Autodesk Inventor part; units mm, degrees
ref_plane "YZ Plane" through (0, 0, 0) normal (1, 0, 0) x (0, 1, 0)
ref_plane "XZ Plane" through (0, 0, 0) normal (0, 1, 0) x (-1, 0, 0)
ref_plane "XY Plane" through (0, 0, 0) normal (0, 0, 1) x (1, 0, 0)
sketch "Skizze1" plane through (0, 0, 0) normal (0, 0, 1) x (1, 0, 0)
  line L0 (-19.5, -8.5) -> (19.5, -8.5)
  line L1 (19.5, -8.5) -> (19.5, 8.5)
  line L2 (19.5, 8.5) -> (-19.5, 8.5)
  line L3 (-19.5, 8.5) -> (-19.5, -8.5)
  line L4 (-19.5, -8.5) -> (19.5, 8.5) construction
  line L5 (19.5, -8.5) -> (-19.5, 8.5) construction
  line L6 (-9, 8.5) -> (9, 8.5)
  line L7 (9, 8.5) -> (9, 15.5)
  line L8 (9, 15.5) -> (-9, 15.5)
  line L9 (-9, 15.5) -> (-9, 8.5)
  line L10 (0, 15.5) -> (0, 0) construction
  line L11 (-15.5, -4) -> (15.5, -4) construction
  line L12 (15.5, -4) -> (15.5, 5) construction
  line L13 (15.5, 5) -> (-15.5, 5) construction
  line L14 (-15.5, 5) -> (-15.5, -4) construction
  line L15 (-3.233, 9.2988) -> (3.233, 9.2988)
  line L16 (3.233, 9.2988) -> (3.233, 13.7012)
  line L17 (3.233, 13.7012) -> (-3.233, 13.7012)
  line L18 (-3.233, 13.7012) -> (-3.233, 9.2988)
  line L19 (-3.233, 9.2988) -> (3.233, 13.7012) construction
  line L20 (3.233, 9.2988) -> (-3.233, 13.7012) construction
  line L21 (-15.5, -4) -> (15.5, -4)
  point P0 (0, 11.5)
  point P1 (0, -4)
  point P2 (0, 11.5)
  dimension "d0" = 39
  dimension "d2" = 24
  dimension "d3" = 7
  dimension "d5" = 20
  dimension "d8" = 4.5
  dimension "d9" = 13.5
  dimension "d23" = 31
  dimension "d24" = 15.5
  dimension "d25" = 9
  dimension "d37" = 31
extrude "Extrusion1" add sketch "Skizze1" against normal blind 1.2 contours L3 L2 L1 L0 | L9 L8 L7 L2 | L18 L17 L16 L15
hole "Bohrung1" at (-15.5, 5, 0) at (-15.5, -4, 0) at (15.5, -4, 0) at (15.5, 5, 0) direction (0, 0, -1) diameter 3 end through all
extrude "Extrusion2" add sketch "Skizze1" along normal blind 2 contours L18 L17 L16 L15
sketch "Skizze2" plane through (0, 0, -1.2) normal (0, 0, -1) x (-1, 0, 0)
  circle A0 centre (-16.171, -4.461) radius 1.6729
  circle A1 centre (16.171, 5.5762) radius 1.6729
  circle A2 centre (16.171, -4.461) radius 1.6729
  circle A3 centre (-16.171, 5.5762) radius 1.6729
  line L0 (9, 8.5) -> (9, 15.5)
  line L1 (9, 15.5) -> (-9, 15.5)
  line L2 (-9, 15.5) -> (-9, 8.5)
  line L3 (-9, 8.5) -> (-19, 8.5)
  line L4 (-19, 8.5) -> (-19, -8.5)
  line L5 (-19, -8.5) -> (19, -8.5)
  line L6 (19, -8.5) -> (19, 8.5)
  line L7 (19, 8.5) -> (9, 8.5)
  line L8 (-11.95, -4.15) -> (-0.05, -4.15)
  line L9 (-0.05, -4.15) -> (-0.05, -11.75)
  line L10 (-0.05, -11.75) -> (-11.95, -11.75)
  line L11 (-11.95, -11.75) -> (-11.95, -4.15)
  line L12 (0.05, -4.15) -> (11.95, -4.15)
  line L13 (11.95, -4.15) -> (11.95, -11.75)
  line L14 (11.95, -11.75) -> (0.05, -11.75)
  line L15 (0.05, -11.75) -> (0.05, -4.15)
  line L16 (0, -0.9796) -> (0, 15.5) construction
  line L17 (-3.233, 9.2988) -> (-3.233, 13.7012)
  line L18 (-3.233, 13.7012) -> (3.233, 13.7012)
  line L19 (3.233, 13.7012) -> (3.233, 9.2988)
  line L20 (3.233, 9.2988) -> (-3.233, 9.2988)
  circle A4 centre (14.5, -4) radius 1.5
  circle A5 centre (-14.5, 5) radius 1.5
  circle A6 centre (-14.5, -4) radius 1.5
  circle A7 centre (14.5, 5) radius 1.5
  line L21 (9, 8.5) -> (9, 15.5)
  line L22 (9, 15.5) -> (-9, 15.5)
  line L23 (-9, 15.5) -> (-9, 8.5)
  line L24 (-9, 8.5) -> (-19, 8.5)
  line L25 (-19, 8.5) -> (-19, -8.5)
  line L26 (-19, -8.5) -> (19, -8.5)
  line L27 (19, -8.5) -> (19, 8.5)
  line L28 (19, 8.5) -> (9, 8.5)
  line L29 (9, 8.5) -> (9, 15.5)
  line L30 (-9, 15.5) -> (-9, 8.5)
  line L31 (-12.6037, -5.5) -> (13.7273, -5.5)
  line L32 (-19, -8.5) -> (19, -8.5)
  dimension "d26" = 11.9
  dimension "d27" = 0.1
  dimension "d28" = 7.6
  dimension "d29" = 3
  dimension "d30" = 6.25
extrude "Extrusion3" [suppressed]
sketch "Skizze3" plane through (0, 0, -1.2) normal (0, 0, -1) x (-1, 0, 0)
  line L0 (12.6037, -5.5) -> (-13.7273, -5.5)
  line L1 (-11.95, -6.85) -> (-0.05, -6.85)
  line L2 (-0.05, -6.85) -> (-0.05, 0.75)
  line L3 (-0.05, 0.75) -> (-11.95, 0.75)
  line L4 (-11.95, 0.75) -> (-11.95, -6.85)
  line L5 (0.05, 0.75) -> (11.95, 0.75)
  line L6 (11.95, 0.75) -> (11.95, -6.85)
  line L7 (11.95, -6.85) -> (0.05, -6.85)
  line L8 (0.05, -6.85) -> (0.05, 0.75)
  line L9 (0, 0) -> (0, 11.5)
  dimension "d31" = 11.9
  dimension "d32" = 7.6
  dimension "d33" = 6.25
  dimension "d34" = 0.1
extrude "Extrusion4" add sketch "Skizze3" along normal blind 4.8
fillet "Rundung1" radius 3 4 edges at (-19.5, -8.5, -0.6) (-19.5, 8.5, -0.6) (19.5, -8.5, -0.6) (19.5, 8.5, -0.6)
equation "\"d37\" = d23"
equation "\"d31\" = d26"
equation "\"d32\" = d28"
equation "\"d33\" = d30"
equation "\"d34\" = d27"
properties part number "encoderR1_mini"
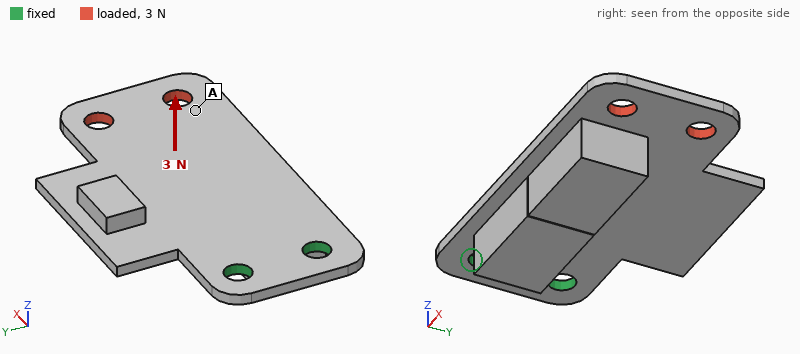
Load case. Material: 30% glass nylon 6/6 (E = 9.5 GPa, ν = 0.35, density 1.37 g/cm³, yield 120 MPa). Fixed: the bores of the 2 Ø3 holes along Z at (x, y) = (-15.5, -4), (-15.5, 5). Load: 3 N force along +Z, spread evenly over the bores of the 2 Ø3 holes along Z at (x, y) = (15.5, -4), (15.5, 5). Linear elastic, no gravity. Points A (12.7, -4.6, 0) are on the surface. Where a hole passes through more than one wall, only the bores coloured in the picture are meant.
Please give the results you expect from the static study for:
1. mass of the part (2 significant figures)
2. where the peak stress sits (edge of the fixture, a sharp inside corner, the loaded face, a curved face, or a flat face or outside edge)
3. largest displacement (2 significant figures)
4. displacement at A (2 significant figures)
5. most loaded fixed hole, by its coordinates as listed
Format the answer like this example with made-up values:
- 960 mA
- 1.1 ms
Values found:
- 2.5 g
- a flat face or outside edge
- 0.51 mm
- 0.38 mm
- (-15.5, 5)
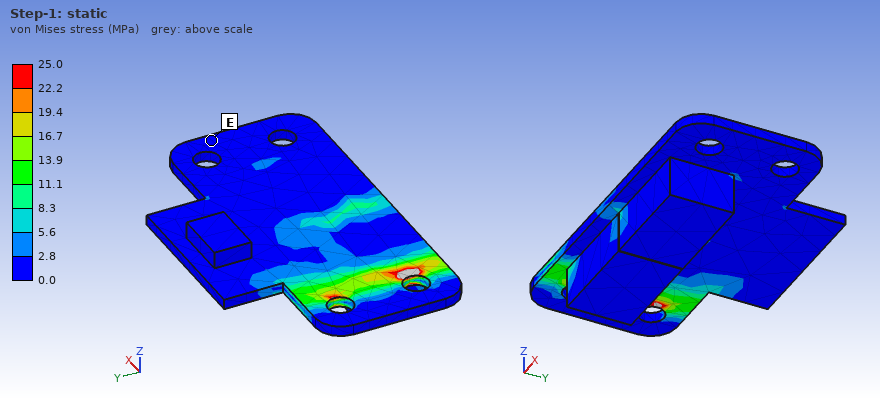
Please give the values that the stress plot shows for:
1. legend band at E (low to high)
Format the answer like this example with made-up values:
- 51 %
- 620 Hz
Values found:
- 0.0 to 2.8 MPa
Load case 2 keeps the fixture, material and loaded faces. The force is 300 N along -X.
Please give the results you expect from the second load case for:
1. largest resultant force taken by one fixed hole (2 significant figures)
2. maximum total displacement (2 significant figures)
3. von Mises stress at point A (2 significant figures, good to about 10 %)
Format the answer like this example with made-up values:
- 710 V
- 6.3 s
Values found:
- 150 N
- 0.19 mm
- 16 MPa
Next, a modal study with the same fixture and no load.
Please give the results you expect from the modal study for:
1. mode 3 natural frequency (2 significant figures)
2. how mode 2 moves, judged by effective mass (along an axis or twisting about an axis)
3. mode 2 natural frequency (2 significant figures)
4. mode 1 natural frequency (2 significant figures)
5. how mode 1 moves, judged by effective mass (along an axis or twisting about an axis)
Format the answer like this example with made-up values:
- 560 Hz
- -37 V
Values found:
- 3600 Hz
- twisting about X
- 2100 Hz
- 510 Hz
- along Z
